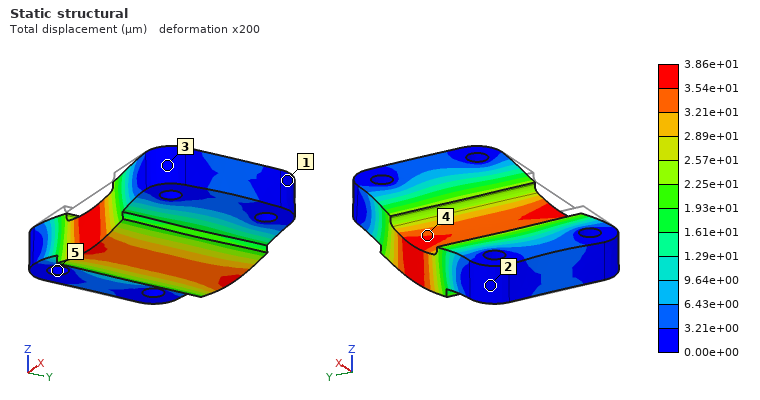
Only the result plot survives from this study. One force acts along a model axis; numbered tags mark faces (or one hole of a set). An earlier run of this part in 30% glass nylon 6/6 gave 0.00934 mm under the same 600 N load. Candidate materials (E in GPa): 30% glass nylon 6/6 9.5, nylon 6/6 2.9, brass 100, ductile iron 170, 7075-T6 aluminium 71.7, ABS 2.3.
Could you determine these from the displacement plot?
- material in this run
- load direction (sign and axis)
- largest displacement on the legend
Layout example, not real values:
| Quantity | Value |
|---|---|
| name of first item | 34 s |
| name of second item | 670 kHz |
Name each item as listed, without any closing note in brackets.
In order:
| Quantity | Value |
|---|---|
| material in this run | ABS |
| load direction | -Z |
| largest displacement on the legend | 3.86e+01 µm |
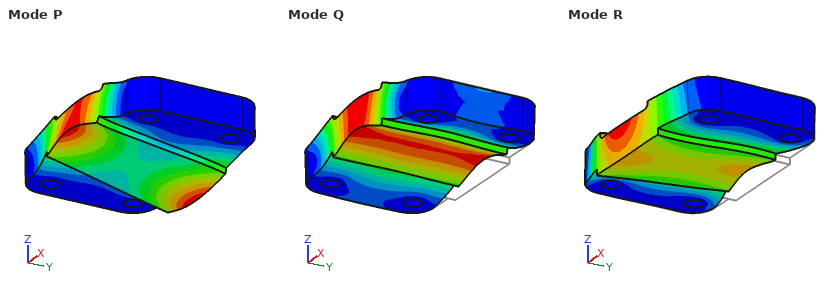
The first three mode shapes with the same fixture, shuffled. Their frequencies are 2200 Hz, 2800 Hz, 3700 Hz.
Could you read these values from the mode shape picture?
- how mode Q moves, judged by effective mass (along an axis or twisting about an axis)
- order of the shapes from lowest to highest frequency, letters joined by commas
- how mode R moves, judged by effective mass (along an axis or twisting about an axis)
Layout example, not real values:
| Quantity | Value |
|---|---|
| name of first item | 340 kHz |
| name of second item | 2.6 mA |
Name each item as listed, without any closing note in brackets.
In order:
| Quantity | Value |
|---|---|
| how mode Q moves, judged by effective mass | along Z |
| order of the shapes from lowest to highest frequency, letters joined by commas | Q, P, R |
| how mode R moves, judged by effective mass | along Y |
